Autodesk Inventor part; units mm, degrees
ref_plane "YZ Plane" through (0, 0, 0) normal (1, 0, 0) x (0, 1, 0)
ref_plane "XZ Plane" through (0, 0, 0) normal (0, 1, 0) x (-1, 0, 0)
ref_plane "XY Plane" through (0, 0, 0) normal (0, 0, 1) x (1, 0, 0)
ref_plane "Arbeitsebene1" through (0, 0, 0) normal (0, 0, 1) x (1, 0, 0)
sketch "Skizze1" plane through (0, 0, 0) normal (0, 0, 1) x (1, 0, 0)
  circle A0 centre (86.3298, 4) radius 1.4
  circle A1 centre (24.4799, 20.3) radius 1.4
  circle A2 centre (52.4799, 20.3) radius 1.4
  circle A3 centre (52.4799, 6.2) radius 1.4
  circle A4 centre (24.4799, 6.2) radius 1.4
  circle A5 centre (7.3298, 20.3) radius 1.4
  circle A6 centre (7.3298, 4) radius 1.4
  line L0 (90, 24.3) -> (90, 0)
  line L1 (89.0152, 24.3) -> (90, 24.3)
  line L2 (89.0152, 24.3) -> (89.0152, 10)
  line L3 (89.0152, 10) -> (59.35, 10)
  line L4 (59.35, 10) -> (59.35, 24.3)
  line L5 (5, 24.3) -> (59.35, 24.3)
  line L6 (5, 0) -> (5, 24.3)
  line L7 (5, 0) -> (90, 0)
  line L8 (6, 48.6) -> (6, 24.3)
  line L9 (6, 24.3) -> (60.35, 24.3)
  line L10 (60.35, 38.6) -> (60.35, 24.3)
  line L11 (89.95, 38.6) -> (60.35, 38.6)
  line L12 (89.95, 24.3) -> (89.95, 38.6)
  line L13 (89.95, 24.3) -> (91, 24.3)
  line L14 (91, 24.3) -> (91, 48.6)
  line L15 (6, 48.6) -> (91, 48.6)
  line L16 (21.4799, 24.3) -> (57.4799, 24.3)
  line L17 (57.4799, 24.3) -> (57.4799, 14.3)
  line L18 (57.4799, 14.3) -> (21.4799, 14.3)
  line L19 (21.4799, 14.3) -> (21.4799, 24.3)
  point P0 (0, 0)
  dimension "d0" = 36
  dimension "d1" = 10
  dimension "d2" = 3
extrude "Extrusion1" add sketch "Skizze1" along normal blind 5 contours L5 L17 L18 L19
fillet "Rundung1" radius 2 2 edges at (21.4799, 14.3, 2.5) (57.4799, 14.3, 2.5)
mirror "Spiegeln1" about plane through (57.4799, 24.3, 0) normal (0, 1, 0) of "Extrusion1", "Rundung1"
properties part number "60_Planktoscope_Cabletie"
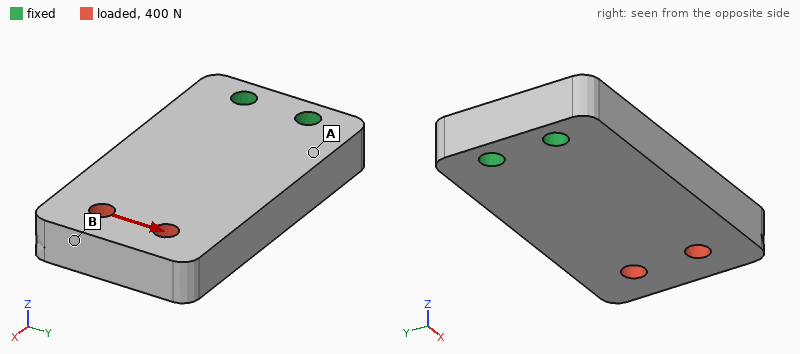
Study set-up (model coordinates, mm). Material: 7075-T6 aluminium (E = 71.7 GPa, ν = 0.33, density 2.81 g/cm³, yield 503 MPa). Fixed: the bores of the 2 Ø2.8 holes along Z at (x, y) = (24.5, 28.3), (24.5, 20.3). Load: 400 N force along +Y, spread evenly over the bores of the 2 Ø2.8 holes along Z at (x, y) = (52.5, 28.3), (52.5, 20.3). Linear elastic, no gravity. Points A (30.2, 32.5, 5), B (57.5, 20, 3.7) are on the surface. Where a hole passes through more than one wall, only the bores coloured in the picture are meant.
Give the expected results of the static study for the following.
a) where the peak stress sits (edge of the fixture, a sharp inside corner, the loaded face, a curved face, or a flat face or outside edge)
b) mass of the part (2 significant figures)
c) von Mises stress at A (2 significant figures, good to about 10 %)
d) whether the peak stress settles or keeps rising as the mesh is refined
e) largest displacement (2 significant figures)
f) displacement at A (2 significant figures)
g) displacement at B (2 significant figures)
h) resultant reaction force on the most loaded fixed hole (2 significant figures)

edge of the fixture
9.7 g
19 MPa
keeps rising
31 µm
5.8 µm
30 µm
1.1 kN
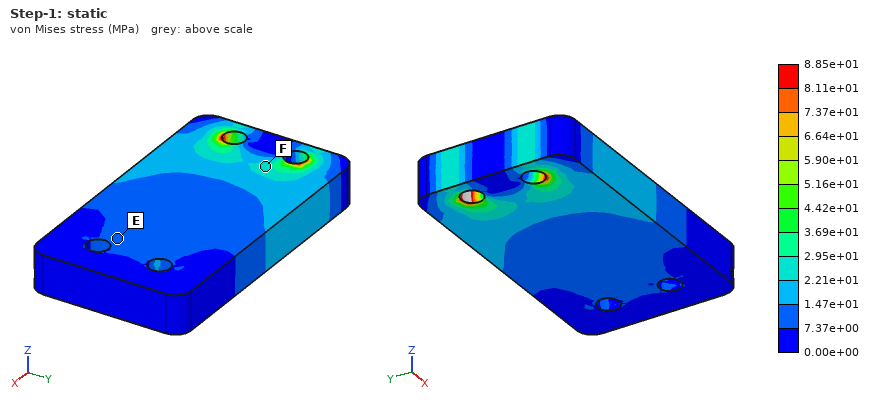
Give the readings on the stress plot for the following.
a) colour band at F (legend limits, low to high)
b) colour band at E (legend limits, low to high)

2.21e+01 to 2.95e+01 MPa
7.37e+00 to 1.47e+01 MPa
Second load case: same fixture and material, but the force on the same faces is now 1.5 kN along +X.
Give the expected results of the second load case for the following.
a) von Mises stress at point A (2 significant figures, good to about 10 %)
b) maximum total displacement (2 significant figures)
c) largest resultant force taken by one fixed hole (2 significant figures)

12 MPa
7.4 µm
750 N
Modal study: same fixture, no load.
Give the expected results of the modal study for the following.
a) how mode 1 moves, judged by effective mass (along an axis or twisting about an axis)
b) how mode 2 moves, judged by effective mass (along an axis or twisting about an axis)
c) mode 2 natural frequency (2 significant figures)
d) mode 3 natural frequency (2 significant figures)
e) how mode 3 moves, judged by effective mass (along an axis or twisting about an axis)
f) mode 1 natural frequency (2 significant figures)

along Z
along Y
10000 Hz
12 kHz
twisting about X
3800 Hz
